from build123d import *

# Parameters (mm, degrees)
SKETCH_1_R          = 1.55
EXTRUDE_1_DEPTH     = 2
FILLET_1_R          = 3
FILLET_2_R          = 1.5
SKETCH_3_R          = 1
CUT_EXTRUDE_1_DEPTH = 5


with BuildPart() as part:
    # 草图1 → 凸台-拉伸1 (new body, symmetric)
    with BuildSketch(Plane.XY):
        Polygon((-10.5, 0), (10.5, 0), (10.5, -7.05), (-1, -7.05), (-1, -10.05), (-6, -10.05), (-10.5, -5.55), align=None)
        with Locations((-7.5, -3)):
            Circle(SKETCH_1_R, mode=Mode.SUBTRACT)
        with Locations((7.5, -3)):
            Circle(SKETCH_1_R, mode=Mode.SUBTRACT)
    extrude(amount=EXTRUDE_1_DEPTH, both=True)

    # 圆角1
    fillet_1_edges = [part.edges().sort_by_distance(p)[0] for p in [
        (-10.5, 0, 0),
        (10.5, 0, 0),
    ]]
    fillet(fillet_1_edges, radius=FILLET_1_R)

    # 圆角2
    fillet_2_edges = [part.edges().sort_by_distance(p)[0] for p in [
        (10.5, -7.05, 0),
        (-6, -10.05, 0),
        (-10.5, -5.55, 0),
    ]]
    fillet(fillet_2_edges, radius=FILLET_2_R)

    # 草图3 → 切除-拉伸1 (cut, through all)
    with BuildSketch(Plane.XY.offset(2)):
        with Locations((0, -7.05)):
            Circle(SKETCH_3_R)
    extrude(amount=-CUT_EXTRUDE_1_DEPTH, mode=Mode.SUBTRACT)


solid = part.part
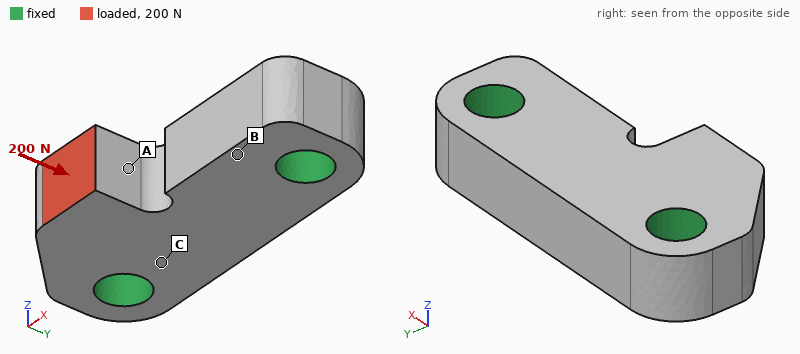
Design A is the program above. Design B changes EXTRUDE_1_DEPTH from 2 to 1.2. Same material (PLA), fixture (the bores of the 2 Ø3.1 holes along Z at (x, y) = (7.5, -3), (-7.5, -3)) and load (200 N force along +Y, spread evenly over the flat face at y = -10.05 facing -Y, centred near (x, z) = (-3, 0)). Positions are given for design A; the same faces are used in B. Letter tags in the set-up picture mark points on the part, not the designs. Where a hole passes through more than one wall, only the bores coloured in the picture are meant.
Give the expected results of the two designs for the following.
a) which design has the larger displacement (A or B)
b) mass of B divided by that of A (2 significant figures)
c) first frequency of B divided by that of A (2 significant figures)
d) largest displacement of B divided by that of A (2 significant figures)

B
0.60
0.72
1.7
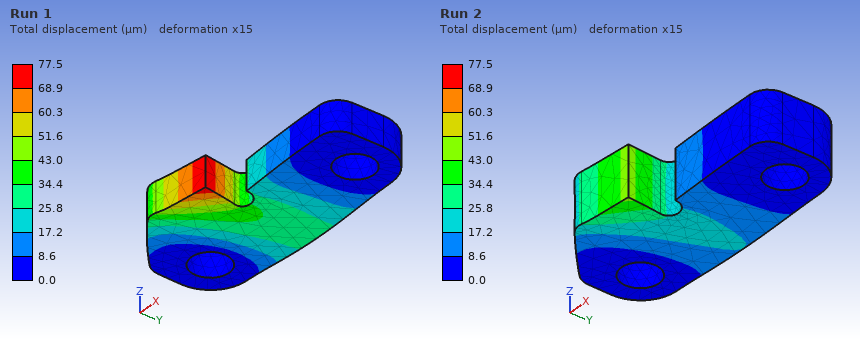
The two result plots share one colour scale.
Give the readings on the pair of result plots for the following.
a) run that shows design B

Run 1
